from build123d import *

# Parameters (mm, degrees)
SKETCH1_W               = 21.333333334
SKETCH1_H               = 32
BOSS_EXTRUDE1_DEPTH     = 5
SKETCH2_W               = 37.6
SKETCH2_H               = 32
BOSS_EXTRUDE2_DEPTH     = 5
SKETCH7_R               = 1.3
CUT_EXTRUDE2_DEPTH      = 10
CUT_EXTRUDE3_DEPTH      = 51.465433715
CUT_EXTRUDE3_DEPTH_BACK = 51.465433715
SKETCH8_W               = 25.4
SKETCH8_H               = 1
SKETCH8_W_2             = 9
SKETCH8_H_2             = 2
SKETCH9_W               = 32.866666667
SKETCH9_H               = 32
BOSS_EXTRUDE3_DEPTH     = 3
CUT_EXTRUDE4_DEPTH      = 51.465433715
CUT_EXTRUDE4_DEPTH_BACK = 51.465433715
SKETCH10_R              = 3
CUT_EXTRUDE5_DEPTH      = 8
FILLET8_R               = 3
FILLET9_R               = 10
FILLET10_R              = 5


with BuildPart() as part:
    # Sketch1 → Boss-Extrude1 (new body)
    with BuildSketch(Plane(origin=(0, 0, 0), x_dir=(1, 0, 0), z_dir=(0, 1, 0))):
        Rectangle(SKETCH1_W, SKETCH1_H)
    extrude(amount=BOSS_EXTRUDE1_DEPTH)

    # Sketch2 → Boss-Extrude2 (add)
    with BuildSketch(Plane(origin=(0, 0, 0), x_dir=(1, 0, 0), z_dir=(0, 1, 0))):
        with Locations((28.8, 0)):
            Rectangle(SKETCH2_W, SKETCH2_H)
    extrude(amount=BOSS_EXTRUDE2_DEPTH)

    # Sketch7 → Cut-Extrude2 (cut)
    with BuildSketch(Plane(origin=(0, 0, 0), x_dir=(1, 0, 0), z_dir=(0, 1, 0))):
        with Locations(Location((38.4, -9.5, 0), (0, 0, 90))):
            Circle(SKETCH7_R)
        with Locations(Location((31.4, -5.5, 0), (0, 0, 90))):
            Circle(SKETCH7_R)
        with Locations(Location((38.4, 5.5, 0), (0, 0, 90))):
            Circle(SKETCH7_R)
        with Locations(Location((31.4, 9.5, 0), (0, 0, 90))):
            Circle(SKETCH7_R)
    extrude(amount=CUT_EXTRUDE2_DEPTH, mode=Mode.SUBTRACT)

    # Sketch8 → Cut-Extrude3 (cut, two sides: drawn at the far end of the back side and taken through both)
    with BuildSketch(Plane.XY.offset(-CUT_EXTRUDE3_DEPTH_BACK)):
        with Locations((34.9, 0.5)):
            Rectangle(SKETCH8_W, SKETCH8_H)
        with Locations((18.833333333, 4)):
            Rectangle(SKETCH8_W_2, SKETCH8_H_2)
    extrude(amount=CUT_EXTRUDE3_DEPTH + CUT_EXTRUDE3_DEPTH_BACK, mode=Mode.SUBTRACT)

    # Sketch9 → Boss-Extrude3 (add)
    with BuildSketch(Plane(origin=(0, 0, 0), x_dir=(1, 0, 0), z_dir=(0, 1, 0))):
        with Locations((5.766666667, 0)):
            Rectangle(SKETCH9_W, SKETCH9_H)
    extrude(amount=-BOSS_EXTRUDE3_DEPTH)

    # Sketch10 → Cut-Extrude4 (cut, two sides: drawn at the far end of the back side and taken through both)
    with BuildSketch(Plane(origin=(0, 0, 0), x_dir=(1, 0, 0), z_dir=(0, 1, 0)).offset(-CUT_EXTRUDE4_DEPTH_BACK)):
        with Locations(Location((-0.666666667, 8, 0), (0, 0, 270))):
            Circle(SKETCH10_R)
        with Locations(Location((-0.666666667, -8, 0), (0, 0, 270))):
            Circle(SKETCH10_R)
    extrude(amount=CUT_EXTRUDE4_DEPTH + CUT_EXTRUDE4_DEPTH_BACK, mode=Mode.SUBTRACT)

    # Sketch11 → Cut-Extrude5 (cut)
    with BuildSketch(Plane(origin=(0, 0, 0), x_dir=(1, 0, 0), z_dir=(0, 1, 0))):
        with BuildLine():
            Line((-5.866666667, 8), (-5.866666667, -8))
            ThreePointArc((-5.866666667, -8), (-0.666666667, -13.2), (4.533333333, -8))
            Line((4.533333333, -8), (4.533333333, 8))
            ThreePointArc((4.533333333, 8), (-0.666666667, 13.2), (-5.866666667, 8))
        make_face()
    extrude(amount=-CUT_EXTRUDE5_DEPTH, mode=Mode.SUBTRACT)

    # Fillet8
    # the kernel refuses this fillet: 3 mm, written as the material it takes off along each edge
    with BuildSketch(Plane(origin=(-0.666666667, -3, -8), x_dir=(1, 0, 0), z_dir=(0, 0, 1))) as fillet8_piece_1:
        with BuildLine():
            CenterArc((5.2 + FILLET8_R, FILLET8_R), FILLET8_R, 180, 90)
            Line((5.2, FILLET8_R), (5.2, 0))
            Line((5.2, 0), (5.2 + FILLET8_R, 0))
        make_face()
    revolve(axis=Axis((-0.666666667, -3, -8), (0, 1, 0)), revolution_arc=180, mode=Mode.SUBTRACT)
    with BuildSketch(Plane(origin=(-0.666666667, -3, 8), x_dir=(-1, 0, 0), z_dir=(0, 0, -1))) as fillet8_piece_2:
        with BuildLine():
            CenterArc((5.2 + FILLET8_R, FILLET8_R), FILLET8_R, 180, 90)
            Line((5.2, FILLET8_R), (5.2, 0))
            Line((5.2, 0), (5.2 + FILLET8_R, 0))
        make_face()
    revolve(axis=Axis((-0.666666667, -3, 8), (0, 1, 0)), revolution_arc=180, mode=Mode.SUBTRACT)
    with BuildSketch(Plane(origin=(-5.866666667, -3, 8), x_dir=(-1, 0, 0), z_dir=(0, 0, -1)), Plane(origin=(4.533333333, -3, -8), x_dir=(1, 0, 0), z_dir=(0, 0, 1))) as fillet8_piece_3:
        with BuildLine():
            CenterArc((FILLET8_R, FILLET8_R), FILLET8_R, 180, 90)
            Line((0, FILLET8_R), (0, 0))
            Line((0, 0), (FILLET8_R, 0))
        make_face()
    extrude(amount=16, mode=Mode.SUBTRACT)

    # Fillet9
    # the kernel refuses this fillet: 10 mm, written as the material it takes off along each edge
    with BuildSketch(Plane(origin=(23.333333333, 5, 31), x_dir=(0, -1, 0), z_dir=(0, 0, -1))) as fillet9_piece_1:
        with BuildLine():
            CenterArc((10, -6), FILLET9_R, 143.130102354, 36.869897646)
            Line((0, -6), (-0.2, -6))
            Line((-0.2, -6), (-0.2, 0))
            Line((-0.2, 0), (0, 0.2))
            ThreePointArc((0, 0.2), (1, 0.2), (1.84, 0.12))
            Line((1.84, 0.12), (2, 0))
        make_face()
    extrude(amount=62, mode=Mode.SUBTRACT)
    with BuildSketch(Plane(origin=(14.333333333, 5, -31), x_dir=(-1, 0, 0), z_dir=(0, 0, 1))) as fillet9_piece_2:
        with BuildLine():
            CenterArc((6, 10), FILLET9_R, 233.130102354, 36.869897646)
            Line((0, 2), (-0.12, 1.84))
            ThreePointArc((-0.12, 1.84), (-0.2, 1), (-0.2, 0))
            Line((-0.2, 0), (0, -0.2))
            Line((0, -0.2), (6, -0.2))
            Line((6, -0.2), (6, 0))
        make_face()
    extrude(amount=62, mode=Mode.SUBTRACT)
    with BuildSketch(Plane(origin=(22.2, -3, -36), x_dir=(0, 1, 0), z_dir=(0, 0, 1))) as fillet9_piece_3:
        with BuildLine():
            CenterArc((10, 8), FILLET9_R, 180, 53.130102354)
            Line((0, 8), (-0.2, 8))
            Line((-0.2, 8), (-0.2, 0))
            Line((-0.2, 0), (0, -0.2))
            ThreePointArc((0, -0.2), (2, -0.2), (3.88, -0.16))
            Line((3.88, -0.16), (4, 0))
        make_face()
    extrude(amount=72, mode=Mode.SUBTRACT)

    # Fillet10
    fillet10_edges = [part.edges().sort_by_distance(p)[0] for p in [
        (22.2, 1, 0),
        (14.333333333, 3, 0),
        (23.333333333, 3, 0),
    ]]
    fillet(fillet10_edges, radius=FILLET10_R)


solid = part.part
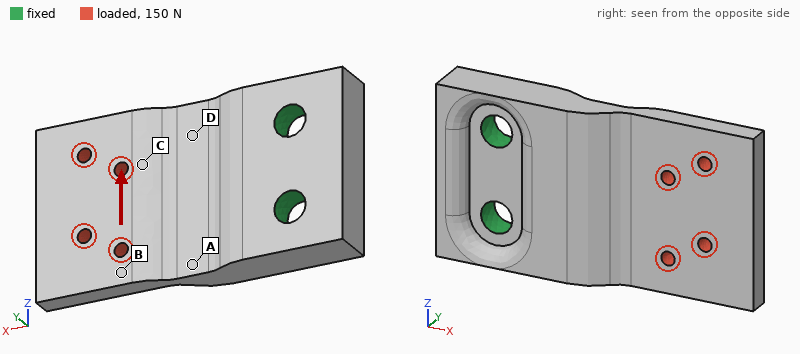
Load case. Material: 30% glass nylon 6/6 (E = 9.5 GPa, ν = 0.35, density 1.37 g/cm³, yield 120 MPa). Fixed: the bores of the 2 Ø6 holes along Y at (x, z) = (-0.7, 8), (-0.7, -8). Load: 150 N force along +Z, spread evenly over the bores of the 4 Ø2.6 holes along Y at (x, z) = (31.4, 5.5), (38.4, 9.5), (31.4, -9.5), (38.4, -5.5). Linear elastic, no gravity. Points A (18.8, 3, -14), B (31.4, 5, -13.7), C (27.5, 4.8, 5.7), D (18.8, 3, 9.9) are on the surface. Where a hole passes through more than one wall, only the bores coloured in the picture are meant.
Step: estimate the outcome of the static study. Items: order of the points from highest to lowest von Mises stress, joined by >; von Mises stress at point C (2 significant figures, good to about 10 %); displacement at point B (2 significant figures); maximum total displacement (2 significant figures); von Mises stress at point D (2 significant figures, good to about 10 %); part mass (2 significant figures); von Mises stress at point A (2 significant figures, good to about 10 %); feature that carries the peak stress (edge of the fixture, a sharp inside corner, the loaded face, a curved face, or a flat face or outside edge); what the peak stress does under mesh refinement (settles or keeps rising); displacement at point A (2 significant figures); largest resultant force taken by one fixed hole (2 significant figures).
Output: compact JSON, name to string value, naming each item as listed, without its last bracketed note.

{"order of the points from highest to lowest von Mises stress, joined by >": "A > D > C > B", "von Mises stress at point C": "2.1 MPa", "displacement at point B": "33 µm", "maximum total displacement": "49 µm", "von Mises stress at point D": "4.4 MPa", "part mass": "13 g", "von Mises stress at point A": "5.6 MPa", "feature that carries the peak stress": "edge of the fixture", "what the peak stress does under mesh refinement": "keeps rising", "displacement at point A": "19 µm", "largest resultant force taken by one fixed hole": "270 N"}
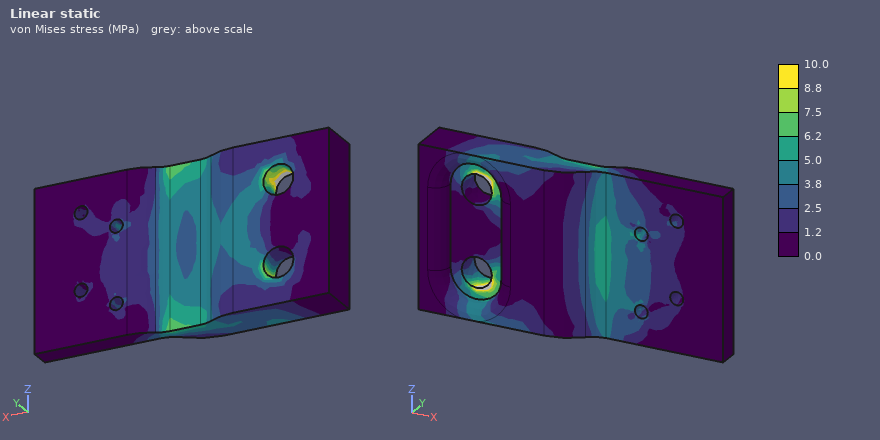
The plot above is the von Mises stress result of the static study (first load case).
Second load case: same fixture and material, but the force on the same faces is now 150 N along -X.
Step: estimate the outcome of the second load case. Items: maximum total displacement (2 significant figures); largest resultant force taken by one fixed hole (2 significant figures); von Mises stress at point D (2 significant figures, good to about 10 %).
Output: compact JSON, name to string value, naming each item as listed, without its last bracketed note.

{"maximum total displacement": "83 µm", "largest resultant force taken by one fixed hole": "76 N", "von Mises stress at point D": "4.4 MPa"}
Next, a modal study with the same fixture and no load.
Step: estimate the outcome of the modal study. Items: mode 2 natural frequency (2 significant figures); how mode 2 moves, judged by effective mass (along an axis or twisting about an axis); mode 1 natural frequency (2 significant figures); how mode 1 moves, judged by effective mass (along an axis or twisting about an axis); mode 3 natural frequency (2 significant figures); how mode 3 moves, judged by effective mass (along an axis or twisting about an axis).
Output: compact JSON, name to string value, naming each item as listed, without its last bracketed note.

{"mode 2 natural frequency": "3000 Hz", "how mode 2 moves, judged by effective mass": "twisting about X", "mode 1 natural frequency": "1100 Hz", "how mode 1 moves, judged by effective mass": "along Y", "mode 3 natural frequency": "4700 Hz", "how mode 3 moves, judged by effective mass": "along Z"}
